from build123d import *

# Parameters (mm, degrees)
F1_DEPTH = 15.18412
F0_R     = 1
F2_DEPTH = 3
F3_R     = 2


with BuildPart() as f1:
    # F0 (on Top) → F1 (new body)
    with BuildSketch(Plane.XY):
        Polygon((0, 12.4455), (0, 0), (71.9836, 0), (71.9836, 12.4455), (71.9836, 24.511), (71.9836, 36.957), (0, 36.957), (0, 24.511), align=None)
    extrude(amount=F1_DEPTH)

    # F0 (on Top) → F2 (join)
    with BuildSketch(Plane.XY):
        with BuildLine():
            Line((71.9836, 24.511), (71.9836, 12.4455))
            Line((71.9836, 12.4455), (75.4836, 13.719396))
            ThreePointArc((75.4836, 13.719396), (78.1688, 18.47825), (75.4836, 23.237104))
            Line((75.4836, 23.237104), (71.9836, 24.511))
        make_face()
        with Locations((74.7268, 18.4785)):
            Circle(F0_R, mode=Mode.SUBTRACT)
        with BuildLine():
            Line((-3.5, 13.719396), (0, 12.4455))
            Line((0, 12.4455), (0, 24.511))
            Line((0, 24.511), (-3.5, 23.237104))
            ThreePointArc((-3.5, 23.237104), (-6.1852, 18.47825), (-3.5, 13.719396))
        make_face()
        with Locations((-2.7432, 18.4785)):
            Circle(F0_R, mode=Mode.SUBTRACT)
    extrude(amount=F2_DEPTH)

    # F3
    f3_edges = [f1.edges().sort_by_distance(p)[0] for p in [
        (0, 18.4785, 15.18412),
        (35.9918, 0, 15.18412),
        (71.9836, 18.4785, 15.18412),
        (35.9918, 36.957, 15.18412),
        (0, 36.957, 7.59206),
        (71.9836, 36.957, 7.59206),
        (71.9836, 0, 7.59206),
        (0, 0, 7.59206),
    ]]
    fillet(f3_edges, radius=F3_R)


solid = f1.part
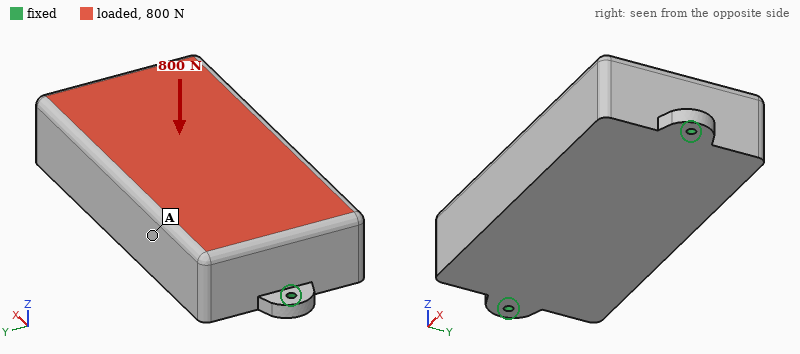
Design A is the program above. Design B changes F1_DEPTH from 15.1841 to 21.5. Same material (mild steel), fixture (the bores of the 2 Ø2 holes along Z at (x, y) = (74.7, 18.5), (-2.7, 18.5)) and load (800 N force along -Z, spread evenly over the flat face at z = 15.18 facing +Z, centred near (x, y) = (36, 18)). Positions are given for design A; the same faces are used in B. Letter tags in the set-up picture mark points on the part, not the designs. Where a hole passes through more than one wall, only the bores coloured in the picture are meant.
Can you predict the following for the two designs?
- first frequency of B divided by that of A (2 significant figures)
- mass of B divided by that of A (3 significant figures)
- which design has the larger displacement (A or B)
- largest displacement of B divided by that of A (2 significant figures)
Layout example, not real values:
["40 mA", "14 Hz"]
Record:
["0.71", "1.41", "A", "0.69"]
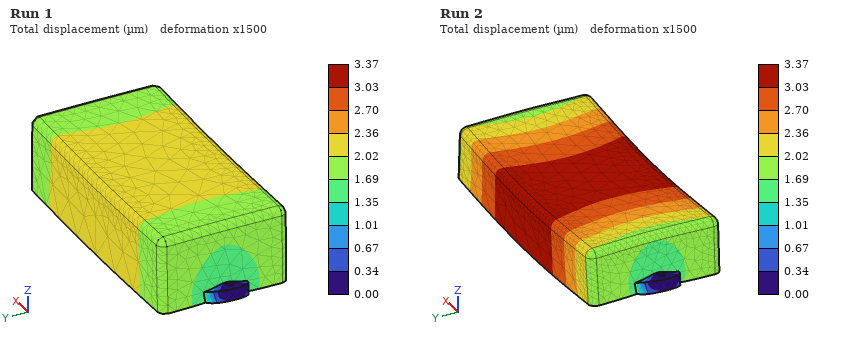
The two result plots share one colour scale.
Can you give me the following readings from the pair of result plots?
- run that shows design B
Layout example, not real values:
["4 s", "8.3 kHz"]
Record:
["Run 1"]
